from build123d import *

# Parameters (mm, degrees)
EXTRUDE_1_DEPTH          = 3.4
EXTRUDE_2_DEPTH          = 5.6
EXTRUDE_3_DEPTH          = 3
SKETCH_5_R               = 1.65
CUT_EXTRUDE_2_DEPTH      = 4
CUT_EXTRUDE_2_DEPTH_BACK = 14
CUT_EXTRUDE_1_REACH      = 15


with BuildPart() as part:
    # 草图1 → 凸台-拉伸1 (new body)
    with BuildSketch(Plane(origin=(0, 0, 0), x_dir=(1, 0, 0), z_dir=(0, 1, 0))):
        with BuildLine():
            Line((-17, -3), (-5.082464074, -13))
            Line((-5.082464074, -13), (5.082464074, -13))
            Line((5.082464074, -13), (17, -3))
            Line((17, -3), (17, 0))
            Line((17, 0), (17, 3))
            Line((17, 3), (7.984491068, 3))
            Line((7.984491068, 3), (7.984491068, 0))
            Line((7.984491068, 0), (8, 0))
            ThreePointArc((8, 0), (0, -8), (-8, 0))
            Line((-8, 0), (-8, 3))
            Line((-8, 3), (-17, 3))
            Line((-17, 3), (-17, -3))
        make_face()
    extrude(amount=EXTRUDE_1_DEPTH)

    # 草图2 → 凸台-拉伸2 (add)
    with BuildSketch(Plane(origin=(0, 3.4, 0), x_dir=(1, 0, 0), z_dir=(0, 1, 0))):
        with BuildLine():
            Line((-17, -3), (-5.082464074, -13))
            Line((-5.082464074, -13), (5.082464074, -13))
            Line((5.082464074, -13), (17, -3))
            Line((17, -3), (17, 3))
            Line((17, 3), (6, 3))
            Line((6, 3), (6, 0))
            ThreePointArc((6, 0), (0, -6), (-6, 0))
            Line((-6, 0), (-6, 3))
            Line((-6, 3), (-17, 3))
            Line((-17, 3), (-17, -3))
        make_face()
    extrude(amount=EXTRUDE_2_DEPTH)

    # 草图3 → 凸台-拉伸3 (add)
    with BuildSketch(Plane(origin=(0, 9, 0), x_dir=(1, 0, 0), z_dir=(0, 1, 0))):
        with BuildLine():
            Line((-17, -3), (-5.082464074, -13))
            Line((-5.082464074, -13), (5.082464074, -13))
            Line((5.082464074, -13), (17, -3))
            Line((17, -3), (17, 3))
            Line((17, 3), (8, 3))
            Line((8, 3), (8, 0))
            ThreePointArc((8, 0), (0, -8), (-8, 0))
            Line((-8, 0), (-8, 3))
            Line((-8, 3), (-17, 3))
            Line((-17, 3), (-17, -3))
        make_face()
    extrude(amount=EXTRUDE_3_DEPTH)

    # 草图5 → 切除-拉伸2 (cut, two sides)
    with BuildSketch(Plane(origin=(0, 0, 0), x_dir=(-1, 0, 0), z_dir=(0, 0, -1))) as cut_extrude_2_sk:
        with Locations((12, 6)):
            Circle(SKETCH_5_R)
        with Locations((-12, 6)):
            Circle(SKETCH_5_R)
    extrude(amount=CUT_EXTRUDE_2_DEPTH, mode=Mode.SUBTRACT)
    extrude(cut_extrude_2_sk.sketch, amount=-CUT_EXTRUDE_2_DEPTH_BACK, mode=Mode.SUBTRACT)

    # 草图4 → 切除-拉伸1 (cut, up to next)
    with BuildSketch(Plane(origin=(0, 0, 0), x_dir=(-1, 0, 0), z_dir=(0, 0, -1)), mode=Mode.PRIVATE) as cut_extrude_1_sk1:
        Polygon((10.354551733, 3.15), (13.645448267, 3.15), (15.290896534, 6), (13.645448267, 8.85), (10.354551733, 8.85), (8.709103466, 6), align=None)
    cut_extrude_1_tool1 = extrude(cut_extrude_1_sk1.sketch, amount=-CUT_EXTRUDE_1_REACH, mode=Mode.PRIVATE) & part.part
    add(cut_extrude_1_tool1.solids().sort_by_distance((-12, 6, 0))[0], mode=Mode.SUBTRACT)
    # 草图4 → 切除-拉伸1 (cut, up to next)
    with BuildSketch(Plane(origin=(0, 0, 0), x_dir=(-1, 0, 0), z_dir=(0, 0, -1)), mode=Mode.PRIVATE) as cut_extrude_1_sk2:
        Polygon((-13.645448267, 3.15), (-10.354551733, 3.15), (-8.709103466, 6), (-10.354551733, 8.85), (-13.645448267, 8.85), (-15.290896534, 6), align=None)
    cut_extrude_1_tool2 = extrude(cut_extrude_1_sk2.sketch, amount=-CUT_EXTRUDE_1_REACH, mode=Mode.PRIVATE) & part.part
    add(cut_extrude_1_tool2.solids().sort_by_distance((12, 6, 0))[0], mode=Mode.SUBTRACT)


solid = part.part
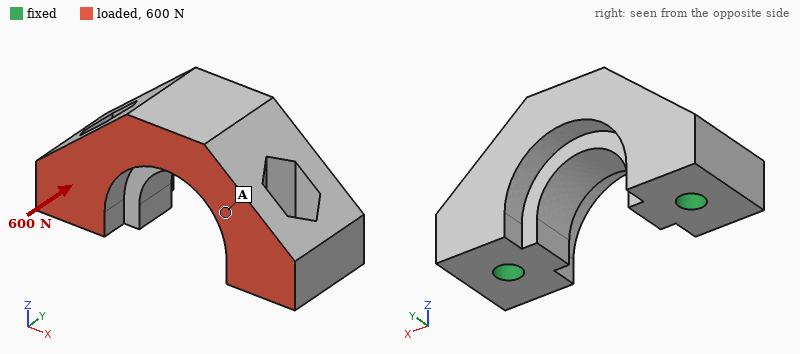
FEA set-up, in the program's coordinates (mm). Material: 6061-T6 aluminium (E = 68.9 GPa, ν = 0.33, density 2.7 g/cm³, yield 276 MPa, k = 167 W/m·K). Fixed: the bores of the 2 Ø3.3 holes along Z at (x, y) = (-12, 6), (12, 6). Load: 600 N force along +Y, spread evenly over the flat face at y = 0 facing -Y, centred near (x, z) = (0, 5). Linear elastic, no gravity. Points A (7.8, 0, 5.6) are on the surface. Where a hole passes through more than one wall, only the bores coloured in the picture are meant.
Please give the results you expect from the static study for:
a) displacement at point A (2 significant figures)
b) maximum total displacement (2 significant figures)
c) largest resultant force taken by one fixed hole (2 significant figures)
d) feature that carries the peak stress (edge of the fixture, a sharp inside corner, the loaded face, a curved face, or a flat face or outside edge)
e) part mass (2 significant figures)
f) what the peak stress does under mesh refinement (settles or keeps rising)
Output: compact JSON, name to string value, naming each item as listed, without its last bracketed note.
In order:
{"displacement at point A": "11 µm", "maximum total displacement": "19 µm", "largest resultant force taken by one fixed hole": "300 N", "feature that carries the peak stress": "edge of the fixture", "part mass": "8.6 g", "what the peak stress does under mesh refinement": "keeps rising"}
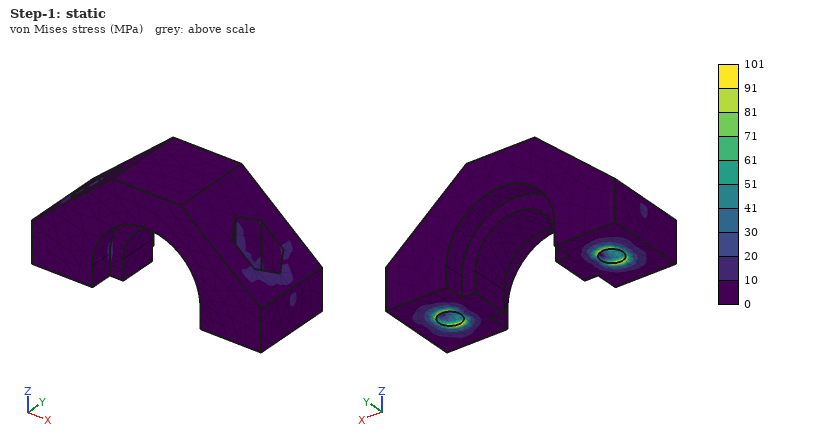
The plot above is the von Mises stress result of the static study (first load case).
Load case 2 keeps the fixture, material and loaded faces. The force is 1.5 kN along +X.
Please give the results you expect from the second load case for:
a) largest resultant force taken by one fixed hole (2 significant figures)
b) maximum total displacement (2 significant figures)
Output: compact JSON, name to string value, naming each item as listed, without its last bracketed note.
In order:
{"largest resultant force taken by one fixed hole": "840 N", "maximum total displacement": "15 µm"}
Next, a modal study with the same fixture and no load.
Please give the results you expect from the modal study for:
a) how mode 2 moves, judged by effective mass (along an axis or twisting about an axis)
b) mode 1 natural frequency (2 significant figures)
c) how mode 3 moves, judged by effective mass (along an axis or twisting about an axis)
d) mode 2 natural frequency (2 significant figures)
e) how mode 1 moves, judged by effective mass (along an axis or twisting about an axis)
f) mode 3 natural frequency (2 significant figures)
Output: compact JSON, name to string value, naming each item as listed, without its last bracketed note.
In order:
{"how mode 2 moves, judged by effective mass": "along X", "mode 1 natural frequency": "11 kHz", "how mode 3 moves, judged by effective mass": "twisting about Z", "mode 2 natural frequency": "26 kHz", "how mode 1 moves, judged by effective mass": "along Y", "mode 3 natural frequency": "29 kHz"}
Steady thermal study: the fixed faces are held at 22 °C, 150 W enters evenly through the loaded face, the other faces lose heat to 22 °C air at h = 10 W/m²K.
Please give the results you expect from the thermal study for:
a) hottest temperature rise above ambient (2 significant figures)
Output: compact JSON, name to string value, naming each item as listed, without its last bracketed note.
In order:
{"hottest temperature rise above ambient": "73 K"}
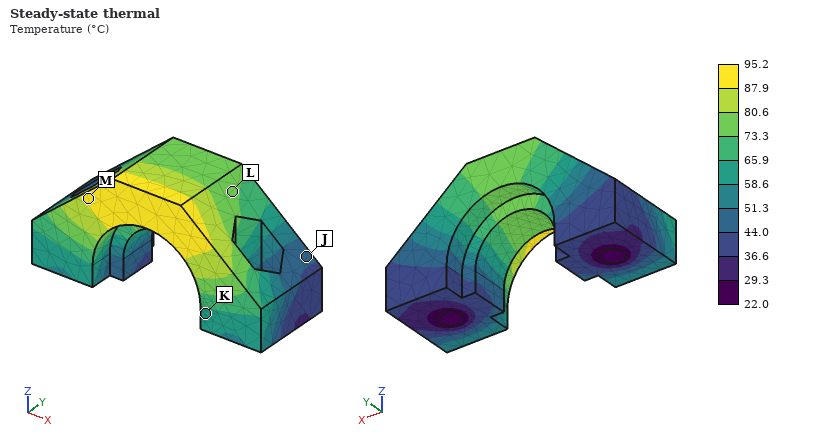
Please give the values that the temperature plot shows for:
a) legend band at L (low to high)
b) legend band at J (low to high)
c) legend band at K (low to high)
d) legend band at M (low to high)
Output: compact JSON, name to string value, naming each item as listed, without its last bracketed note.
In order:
{"legend band at L": "73.3 to 80.6 °C", "legend band at J": "44.0 to 51.3 °C", "legend band at K": "58.6 to 65.9 °C", "legend band at M": "87.9 to 95.2 °C"}
